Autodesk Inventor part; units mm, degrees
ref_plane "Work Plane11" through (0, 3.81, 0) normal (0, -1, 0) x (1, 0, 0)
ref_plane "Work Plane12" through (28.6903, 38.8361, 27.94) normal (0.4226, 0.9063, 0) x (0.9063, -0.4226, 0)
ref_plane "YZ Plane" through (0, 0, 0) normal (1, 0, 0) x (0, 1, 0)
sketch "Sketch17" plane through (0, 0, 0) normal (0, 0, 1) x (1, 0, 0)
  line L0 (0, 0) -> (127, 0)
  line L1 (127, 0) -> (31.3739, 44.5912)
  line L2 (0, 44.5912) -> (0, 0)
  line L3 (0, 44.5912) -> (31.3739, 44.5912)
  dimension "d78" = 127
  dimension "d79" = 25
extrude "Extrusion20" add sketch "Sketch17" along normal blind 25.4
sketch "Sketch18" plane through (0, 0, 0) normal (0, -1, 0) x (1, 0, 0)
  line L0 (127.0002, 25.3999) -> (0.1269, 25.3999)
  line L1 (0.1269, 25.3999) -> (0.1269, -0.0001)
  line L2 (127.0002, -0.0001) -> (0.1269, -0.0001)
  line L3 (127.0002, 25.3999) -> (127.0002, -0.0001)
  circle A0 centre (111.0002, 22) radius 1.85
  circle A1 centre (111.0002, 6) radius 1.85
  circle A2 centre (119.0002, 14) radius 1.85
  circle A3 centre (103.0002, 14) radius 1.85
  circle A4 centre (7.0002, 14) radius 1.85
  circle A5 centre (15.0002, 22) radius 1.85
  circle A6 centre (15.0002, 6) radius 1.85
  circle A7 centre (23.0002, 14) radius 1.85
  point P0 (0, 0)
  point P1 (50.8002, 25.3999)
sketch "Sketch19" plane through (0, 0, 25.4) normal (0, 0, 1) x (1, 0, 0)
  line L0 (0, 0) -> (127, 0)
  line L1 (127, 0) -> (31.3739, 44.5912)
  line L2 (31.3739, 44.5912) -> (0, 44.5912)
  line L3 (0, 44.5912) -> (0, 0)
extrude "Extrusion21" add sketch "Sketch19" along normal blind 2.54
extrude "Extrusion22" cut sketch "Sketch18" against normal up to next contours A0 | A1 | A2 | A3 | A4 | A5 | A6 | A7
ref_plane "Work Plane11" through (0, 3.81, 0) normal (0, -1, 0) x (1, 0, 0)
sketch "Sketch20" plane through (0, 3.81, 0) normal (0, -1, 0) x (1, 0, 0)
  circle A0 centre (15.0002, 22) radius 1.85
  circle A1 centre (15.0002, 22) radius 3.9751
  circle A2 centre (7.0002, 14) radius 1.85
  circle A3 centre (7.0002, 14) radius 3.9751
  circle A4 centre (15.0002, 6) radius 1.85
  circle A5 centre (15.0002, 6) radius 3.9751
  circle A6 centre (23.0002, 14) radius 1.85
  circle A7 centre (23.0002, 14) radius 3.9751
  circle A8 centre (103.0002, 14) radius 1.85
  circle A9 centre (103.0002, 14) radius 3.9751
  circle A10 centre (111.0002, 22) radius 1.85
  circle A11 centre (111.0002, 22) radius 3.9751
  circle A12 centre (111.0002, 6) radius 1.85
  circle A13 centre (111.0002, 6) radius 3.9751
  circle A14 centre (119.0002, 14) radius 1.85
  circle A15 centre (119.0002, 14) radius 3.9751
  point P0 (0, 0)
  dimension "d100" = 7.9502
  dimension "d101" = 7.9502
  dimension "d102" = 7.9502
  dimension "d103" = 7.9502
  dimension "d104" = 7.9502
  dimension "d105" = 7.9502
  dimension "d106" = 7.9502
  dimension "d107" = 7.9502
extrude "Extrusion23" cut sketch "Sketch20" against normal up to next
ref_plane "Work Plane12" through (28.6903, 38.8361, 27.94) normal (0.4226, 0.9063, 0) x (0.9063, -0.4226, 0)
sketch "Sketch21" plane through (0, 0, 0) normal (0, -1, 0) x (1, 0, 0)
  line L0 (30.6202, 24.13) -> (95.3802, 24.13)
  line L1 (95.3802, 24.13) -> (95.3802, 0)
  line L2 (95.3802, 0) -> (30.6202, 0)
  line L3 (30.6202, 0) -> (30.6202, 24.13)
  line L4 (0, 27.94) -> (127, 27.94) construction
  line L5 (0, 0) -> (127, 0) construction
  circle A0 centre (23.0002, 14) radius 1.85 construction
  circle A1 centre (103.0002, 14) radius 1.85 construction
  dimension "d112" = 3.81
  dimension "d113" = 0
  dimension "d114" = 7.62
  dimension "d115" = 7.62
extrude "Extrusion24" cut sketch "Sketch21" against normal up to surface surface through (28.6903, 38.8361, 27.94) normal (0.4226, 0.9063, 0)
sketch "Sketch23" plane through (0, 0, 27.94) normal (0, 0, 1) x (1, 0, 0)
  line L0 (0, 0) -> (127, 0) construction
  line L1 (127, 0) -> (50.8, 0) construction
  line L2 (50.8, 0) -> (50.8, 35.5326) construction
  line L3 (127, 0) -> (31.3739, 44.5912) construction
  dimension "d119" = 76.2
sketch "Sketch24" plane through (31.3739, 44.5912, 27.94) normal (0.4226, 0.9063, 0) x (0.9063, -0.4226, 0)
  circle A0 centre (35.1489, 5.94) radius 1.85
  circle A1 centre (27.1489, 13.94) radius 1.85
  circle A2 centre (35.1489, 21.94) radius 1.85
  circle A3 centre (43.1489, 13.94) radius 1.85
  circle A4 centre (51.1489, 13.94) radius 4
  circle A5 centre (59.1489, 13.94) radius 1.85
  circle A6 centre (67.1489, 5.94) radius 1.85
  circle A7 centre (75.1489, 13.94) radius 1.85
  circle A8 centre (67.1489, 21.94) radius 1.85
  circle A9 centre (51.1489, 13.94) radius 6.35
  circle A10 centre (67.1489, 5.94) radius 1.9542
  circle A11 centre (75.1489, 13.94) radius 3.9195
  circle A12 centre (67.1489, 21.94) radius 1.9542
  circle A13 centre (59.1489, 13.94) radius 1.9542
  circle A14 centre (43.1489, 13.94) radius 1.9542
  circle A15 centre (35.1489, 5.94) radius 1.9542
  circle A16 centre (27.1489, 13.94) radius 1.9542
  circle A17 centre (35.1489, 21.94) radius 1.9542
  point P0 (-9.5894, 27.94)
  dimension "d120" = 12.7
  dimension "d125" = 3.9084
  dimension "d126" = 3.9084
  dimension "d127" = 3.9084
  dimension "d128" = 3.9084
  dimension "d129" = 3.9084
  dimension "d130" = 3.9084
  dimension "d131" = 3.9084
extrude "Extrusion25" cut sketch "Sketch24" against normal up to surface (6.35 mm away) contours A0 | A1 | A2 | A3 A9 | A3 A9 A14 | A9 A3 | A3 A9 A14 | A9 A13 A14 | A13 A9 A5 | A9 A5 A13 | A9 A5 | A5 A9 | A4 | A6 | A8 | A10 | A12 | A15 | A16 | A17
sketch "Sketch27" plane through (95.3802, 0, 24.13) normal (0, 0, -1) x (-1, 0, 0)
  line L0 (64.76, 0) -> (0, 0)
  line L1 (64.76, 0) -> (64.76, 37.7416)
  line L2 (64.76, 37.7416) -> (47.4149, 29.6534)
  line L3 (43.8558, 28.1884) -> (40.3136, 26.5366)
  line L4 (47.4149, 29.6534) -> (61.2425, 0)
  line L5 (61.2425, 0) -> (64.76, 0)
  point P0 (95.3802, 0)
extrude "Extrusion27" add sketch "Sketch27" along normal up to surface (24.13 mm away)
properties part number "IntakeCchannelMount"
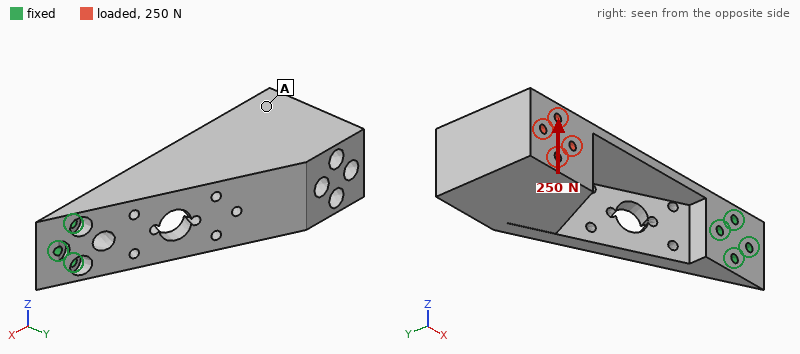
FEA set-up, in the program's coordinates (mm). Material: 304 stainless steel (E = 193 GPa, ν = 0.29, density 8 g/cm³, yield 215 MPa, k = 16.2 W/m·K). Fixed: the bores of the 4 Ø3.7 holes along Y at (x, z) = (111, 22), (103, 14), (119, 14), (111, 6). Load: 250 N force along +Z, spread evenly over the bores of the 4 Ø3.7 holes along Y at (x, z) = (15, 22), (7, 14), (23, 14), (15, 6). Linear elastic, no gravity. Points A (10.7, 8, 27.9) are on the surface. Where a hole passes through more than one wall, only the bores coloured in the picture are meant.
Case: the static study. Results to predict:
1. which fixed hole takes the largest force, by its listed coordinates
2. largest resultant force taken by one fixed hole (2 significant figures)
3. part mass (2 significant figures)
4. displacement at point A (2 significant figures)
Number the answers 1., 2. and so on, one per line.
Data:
1. (103, 14)
2. 1.1 kN
3. 490 g
4. 0.21 mm
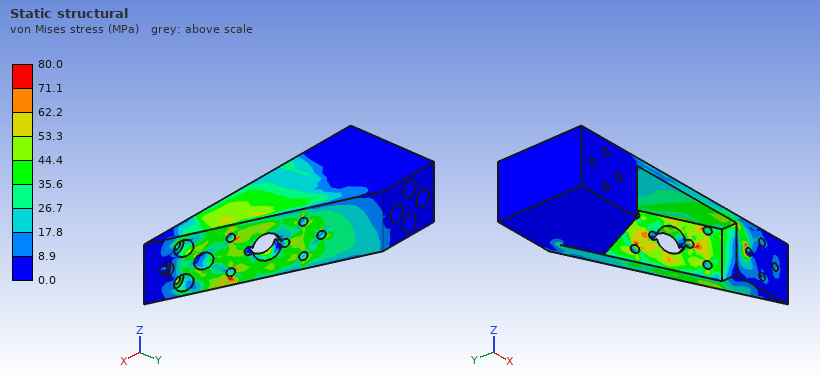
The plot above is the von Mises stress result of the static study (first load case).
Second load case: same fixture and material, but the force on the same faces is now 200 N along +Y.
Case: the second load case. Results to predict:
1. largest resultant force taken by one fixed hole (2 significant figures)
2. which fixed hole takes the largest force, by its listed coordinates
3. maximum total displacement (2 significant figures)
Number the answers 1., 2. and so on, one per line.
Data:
1. 1.6 kN
2. (103, 14)
3. 0.18 mm
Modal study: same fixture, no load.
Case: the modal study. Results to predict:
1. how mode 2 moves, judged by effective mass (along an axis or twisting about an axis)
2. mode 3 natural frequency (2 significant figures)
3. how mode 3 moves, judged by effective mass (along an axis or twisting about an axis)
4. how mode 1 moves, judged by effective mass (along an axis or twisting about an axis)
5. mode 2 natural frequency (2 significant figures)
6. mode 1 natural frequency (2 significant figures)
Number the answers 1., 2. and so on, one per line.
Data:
1. along Z
2. 1400 Hz
3. along Z
4. along Y
5. 450 Hz
6. 320 Hz
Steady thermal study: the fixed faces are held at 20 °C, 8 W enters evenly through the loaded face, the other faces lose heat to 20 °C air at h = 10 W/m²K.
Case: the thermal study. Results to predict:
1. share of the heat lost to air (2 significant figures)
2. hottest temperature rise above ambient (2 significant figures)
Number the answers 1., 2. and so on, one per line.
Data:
1. 84 %
2. 60 K
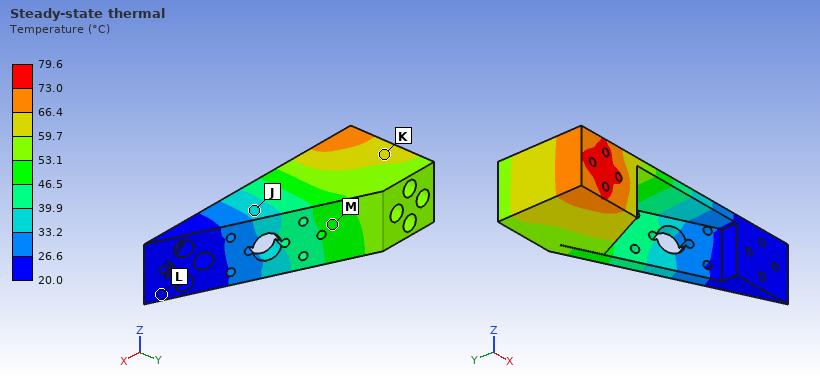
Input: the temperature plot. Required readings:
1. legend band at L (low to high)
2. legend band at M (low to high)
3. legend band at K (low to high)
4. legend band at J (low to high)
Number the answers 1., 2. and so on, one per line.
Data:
1. 20.0 to 26.6 °C
2. 46.5 to 53.1 °C
3. 59.7 to 66.4 °C
4. 33.2 to 39.9 °C
